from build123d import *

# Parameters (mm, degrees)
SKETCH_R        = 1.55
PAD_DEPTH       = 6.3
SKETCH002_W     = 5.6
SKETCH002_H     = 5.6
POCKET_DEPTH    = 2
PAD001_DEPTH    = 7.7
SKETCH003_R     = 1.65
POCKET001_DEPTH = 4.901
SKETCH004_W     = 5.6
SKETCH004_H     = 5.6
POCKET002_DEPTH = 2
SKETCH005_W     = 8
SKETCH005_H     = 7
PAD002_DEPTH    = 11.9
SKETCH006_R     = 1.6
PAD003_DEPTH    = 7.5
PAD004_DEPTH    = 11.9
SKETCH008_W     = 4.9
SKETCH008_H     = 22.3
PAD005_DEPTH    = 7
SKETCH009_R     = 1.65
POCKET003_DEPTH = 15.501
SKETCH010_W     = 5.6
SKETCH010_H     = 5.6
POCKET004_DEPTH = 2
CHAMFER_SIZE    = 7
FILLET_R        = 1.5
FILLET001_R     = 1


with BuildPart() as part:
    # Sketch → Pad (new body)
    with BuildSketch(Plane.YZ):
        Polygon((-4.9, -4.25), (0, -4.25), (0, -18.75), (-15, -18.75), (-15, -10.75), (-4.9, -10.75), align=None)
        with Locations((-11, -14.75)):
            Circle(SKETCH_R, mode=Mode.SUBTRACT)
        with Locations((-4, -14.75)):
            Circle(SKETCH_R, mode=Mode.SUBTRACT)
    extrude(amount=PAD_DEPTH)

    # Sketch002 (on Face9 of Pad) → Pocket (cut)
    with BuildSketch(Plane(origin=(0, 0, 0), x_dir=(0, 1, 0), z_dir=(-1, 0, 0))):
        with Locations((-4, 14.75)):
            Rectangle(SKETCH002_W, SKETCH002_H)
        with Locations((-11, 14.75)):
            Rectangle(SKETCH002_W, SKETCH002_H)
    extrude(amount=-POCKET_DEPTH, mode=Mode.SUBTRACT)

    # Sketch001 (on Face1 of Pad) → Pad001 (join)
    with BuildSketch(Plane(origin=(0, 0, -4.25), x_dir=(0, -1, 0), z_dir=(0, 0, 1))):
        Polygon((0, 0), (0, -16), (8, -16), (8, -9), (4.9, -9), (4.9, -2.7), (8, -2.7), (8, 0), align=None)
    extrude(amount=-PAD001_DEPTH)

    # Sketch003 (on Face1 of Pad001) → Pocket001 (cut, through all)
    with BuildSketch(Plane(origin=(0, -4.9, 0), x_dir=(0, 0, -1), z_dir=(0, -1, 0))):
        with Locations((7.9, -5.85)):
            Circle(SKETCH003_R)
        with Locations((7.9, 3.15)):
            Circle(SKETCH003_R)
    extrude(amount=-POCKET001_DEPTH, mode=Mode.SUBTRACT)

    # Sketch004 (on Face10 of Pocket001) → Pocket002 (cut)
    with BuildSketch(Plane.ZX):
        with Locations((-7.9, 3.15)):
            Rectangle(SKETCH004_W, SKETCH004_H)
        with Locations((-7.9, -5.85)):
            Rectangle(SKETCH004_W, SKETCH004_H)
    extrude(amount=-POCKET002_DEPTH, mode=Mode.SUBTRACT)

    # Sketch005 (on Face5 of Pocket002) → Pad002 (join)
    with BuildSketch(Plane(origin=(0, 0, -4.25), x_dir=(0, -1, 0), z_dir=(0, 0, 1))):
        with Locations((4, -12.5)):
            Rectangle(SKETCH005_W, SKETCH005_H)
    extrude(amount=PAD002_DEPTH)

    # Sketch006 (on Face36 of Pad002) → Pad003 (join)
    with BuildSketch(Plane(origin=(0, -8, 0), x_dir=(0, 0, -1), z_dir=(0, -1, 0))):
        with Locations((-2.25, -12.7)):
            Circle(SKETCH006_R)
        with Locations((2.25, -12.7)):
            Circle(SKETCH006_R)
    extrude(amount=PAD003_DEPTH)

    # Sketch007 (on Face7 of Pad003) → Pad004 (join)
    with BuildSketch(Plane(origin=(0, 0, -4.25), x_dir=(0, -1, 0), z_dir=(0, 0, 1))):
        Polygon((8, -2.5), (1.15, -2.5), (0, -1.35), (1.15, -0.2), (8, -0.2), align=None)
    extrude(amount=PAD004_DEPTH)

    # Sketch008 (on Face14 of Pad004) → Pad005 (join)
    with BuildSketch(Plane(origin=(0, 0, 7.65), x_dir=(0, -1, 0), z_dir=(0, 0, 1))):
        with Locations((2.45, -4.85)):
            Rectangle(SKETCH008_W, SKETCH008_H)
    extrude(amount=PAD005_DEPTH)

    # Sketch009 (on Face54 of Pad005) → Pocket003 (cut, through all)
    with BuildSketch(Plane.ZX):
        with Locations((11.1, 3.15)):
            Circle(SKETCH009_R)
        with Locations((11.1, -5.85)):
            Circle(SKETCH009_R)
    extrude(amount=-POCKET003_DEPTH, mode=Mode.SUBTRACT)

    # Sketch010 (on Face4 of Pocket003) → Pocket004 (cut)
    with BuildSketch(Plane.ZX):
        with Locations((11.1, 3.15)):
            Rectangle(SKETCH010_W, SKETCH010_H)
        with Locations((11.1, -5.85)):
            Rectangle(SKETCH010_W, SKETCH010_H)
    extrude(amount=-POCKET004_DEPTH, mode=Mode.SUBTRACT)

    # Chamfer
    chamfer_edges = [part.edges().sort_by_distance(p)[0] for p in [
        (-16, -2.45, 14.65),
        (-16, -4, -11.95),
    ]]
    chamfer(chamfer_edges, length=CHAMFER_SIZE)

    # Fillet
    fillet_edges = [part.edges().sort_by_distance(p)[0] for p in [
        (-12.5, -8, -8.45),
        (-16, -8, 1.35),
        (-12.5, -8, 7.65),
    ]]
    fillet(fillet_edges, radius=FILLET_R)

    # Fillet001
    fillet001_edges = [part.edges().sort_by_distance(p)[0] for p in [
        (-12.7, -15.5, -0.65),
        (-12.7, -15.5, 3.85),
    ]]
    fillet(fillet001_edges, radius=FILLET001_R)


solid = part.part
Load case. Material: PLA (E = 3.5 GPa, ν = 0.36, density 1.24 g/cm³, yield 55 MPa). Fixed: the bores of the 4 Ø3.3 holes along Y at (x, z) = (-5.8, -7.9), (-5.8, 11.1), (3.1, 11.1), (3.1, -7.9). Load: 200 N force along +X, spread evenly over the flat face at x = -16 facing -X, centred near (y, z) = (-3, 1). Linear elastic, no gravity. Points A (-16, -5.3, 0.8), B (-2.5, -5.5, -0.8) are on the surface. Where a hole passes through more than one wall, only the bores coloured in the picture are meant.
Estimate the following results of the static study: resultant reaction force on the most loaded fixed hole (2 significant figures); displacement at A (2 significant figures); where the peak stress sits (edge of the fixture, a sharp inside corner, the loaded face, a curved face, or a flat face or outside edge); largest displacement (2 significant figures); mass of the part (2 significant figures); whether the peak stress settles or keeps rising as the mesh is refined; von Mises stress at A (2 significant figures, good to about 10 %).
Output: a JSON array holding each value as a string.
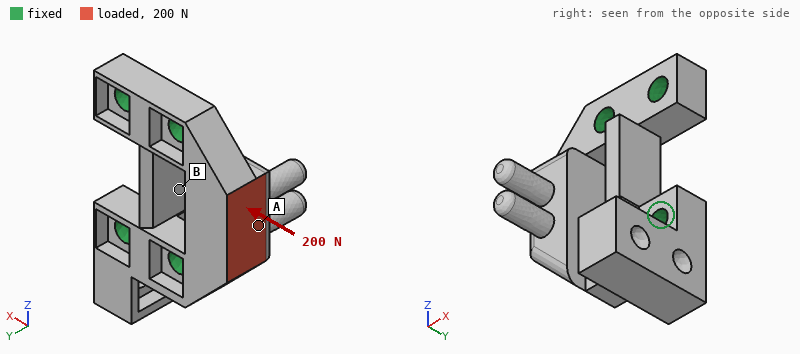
["110 N", "24 µm", "a sharp inside corner", "33 µm", "3.3 g", "keeps rising", "3.9 MPa"]
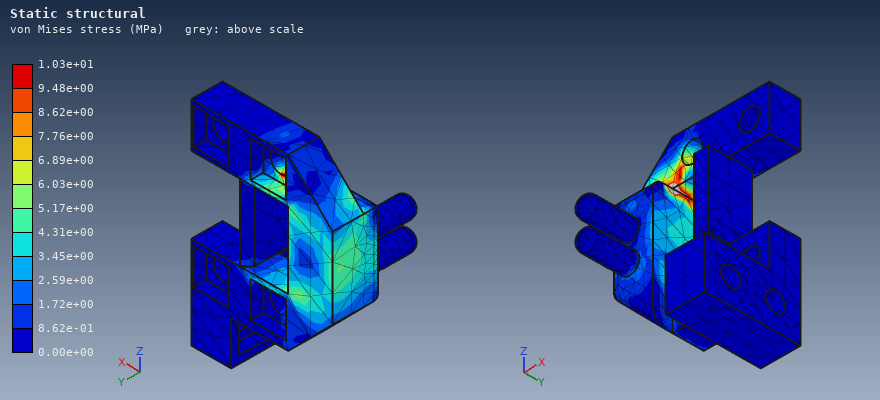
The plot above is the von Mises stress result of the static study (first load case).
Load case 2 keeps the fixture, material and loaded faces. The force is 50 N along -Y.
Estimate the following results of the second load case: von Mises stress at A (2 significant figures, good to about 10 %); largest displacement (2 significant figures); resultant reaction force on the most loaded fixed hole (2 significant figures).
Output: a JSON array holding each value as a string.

["1.3 MPa", "0.14 mm", "35 N"]
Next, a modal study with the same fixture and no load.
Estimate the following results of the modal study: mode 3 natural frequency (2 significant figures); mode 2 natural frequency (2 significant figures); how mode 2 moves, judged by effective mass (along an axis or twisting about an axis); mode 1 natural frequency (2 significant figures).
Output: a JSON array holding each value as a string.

["6100 Hz", "4500 Hz", "along Y", "3800 Hz"]
